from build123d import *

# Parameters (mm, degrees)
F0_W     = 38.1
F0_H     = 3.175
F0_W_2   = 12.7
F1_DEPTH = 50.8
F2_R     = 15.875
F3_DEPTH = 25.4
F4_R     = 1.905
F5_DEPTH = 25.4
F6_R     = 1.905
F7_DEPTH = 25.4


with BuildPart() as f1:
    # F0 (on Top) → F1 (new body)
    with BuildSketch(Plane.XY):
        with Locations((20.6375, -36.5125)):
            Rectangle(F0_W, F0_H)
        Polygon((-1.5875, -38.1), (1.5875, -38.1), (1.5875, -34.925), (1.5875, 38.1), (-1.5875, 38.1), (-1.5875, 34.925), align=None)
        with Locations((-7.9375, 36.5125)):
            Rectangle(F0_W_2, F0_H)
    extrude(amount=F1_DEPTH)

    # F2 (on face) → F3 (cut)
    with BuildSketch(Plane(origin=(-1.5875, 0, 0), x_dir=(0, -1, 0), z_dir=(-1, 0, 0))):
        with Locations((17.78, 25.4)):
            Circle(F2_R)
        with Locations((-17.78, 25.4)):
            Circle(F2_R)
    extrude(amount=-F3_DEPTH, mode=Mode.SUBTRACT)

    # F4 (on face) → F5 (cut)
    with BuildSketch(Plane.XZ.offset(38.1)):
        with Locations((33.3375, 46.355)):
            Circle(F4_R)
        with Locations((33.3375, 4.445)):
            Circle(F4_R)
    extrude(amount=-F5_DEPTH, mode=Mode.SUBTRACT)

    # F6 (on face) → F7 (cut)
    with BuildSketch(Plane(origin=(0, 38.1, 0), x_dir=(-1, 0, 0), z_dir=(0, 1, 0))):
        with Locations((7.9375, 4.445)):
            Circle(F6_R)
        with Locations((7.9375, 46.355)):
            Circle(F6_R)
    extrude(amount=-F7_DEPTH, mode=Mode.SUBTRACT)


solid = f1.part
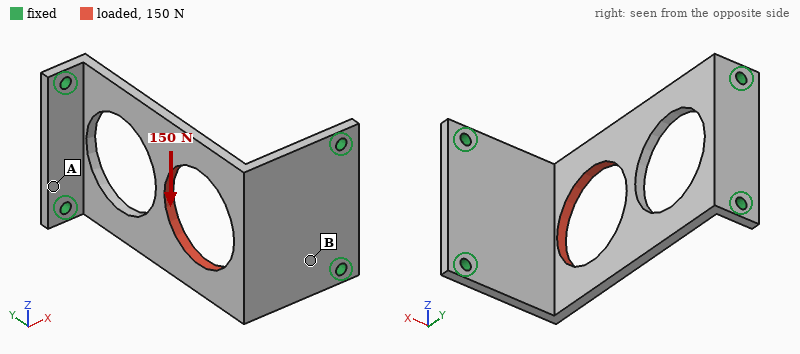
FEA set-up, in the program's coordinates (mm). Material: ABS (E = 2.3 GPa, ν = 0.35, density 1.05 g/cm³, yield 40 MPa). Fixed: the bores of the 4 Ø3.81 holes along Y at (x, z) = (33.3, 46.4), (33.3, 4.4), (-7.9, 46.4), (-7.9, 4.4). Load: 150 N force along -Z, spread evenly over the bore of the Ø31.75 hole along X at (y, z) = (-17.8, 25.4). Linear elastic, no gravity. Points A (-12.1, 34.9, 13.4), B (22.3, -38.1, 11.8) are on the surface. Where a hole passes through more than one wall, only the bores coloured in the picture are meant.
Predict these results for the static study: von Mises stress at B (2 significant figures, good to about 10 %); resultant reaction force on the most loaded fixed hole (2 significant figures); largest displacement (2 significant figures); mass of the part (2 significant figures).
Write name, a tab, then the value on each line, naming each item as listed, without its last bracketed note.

von Mises stress at B	1.5 MPa
resultant reaction force on the most loaded fixed hole	100 N
largest displacement	0.14 mm
mass of the part	16 g
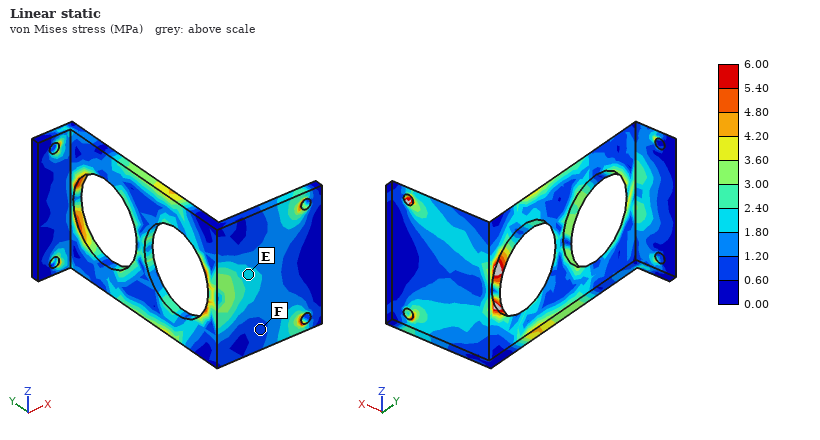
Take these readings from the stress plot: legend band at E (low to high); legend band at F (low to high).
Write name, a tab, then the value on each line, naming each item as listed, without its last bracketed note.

legend band at E	1.80 to 2.40 MPa
legend band at F	0.60 to 1.20 MPa
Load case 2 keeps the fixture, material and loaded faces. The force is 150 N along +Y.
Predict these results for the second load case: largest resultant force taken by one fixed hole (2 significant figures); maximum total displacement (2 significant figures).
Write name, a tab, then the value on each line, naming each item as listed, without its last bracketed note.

largest resultant force taken by one fixed hole	74 N
maximum total displacement	0.28 mm
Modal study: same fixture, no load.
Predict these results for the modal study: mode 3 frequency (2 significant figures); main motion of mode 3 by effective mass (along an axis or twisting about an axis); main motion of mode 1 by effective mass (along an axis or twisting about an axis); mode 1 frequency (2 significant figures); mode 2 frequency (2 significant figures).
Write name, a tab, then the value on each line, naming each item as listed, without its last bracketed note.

mode 3 frequency	1700 Hz
main motion of mode 3 by effective mass	along Y
main motion of mode 1 by effective mass	along X
mode 1 frequency	690 Hz
mode 2 frequency	940 Hz
